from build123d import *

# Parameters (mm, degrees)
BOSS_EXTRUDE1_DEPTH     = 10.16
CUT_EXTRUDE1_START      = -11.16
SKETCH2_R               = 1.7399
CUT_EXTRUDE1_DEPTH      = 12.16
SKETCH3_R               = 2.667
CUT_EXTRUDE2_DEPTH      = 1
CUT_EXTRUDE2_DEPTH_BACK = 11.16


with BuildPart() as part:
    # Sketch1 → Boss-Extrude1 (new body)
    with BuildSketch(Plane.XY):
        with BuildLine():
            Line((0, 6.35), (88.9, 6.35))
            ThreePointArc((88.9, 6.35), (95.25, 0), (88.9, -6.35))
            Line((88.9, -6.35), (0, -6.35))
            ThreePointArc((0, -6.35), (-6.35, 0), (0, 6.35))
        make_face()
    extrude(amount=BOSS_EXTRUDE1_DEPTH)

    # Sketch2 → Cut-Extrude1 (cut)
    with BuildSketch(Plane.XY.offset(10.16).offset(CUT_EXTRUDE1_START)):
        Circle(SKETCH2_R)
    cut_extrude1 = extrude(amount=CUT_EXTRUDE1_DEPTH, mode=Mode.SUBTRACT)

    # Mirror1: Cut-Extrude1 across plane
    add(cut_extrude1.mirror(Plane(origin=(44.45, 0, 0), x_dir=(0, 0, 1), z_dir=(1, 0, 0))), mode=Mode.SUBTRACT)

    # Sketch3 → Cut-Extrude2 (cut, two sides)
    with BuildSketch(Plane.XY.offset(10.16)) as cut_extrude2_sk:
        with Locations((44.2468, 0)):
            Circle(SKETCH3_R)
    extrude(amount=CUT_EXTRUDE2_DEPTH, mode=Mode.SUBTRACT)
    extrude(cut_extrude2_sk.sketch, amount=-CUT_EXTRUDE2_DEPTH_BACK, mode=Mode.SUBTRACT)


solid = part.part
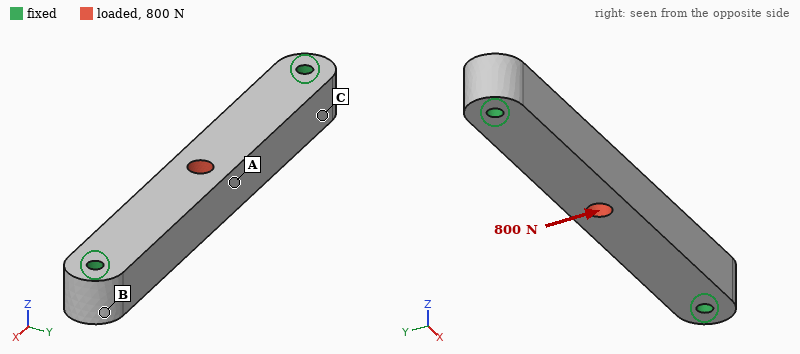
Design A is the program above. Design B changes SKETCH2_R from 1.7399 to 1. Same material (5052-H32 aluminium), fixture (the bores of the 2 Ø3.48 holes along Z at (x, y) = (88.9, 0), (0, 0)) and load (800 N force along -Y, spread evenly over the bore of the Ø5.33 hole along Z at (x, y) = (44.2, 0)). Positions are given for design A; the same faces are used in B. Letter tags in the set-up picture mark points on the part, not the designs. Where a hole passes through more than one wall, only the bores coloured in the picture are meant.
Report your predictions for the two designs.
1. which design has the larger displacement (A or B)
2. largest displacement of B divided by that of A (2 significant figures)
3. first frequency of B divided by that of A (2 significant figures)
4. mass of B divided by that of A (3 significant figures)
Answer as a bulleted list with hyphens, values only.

- B
- 1.4
- 0.81
- 1.01
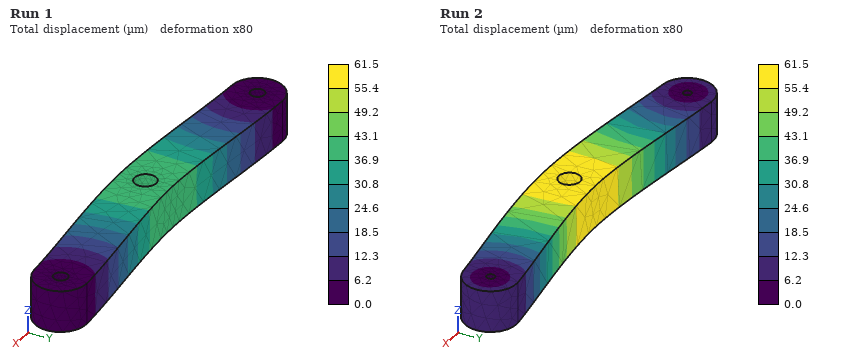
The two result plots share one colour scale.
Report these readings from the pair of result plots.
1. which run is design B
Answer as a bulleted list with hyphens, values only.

- Run 2
